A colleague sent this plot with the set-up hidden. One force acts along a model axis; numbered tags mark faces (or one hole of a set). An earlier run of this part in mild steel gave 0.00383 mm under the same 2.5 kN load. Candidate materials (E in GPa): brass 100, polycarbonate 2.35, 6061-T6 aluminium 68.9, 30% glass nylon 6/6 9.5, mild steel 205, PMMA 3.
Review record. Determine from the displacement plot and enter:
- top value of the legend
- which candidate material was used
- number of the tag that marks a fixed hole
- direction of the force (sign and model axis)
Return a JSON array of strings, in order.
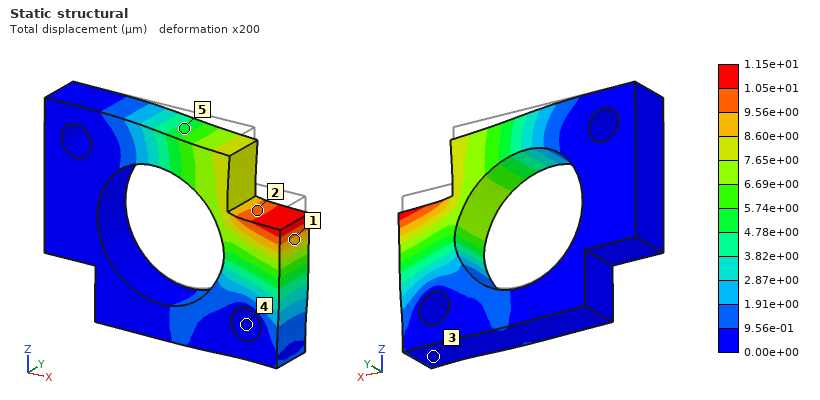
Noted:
["1.15e+01 µm", "6061-T6 aluminium", "4", "-Z"]
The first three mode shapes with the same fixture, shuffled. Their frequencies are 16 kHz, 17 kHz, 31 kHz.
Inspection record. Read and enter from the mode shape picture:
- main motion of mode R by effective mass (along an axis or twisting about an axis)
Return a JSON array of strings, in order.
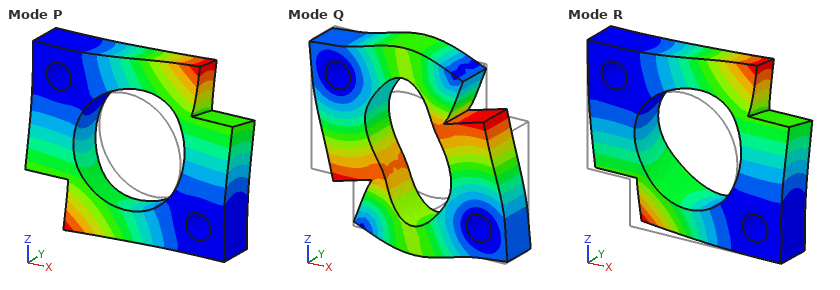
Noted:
["along Y"]
